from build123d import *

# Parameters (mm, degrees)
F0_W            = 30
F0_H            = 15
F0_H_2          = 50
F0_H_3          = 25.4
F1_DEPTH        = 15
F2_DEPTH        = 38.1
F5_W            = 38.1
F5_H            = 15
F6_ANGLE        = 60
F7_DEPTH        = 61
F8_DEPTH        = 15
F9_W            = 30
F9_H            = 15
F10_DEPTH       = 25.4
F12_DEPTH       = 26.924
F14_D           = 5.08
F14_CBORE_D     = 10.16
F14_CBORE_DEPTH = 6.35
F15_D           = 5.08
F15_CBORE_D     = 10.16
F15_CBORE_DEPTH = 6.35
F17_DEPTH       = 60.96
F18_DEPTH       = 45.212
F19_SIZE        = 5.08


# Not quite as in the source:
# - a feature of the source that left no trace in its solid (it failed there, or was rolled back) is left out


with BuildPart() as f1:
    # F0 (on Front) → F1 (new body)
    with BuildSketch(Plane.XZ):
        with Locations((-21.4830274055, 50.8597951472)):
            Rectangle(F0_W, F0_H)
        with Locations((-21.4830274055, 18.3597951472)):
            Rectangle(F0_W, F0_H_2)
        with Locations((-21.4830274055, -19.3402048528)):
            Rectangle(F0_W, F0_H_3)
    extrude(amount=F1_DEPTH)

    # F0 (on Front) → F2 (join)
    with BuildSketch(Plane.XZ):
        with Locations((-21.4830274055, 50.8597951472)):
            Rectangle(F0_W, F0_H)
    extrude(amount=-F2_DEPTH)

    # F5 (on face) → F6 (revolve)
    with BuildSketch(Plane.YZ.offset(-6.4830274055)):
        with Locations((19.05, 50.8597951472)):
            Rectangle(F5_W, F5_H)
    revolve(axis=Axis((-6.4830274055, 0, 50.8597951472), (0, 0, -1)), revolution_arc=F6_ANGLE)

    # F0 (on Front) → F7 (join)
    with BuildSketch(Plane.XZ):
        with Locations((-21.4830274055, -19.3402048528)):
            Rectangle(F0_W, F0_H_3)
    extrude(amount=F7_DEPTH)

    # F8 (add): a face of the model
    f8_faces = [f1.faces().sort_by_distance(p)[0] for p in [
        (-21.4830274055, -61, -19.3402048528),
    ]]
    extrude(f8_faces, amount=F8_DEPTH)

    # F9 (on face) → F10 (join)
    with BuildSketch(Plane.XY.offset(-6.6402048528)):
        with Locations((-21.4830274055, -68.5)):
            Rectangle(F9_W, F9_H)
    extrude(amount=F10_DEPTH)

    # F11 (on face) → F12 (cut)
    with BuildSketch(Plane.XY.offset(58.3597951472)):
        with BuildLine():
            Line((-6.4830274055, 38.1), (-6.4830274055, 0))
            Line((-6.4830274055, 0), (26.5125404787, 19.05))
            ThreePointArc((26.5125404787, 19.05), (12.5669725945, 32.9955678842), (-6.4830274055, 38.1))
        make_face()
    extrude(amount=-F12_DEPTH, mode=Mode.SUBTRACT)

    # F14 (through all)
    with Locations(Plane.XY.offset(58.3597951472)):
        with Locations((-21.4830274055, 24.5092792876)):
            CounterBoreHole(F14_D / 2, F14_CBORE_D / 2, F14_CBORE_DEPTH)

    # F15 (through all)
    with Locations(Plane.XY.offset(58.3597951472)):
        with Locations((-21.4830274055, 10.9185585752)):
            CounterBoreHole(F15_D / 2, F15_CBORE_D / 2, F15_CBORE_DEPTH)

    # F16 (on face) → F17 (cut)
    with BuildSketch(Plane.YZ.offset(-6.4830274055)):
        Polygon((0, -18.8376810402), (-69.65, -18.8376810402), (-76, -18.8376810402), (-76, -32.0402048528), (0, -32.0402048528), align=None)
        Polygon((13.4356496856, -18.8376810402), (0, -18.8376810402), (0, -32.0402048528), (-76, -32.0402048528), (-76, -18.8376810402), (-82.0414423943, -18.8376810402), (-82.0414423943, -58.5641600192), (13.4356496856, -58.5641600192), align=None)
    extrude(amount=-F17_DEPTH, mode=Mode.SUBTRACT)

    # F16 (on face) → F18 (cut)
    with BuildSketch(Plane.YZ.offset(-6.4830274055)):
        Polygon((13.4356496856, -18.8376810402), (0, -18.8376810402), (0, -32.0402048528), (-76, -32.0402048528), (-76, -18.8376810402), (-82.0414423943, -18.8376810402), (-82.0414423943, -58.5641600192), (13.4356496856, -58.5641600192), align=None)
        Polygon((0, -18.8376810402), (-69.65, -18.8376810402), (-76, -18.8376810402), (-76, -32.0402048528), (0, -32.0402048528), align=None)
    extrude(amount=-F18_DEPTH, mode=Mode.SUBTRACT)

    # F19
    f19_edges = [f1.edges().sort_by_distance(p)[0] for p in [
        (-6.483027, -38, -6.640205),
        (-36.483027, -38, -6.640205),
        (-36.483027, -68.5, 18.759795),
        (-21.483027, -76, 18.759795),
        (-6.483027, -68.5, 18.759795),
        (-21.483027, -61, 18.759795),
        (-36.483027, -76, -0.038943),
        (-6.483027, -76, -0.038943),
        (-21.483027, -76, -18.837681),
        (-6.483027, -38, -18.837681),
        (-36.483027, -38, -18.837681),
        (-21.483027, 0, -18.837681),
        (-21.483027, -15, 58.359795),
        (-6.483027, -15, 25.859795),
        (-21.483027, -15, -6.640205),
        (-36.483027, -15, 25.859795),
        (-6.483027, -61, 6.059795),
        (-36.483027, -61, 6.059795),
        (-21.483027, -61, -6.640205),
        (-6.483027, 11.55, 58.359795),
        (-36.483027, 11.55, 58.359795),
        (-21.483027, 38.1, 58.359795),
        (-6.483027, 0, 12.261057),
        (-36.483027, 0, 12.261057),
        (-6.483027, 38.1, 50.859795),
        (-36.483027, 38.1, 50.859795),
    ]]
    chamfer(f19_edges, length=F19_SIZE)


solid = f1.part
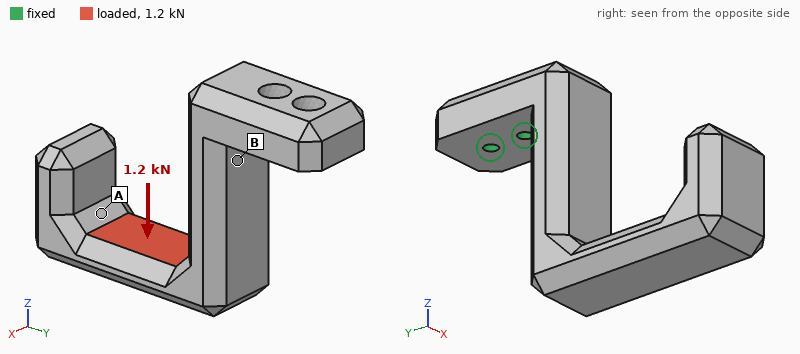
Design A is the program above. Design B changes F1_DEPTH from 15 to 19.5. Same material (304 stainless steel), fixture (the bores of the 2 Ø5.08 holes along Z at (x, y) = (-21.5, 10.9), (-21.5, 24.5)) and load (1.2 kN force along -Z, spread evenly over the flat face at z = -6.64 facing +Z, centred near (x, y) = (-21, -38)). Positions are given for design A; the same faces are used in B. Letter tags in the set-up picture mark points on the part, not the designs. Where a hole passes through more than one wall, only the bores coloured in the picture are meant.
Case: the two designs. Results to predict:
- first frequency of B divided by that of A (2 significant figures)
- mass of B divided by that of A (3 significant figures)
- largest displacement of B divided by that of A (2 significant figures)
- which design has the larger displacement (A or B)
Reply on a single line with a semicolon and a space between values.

1.2; 1.12; 0.73; A
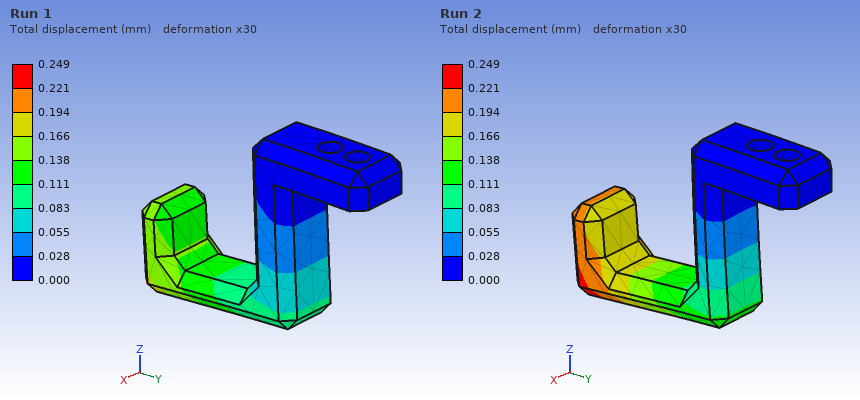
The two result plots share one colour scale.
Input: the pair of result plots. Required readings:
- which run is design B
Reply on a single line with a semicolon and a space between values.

Run 1
